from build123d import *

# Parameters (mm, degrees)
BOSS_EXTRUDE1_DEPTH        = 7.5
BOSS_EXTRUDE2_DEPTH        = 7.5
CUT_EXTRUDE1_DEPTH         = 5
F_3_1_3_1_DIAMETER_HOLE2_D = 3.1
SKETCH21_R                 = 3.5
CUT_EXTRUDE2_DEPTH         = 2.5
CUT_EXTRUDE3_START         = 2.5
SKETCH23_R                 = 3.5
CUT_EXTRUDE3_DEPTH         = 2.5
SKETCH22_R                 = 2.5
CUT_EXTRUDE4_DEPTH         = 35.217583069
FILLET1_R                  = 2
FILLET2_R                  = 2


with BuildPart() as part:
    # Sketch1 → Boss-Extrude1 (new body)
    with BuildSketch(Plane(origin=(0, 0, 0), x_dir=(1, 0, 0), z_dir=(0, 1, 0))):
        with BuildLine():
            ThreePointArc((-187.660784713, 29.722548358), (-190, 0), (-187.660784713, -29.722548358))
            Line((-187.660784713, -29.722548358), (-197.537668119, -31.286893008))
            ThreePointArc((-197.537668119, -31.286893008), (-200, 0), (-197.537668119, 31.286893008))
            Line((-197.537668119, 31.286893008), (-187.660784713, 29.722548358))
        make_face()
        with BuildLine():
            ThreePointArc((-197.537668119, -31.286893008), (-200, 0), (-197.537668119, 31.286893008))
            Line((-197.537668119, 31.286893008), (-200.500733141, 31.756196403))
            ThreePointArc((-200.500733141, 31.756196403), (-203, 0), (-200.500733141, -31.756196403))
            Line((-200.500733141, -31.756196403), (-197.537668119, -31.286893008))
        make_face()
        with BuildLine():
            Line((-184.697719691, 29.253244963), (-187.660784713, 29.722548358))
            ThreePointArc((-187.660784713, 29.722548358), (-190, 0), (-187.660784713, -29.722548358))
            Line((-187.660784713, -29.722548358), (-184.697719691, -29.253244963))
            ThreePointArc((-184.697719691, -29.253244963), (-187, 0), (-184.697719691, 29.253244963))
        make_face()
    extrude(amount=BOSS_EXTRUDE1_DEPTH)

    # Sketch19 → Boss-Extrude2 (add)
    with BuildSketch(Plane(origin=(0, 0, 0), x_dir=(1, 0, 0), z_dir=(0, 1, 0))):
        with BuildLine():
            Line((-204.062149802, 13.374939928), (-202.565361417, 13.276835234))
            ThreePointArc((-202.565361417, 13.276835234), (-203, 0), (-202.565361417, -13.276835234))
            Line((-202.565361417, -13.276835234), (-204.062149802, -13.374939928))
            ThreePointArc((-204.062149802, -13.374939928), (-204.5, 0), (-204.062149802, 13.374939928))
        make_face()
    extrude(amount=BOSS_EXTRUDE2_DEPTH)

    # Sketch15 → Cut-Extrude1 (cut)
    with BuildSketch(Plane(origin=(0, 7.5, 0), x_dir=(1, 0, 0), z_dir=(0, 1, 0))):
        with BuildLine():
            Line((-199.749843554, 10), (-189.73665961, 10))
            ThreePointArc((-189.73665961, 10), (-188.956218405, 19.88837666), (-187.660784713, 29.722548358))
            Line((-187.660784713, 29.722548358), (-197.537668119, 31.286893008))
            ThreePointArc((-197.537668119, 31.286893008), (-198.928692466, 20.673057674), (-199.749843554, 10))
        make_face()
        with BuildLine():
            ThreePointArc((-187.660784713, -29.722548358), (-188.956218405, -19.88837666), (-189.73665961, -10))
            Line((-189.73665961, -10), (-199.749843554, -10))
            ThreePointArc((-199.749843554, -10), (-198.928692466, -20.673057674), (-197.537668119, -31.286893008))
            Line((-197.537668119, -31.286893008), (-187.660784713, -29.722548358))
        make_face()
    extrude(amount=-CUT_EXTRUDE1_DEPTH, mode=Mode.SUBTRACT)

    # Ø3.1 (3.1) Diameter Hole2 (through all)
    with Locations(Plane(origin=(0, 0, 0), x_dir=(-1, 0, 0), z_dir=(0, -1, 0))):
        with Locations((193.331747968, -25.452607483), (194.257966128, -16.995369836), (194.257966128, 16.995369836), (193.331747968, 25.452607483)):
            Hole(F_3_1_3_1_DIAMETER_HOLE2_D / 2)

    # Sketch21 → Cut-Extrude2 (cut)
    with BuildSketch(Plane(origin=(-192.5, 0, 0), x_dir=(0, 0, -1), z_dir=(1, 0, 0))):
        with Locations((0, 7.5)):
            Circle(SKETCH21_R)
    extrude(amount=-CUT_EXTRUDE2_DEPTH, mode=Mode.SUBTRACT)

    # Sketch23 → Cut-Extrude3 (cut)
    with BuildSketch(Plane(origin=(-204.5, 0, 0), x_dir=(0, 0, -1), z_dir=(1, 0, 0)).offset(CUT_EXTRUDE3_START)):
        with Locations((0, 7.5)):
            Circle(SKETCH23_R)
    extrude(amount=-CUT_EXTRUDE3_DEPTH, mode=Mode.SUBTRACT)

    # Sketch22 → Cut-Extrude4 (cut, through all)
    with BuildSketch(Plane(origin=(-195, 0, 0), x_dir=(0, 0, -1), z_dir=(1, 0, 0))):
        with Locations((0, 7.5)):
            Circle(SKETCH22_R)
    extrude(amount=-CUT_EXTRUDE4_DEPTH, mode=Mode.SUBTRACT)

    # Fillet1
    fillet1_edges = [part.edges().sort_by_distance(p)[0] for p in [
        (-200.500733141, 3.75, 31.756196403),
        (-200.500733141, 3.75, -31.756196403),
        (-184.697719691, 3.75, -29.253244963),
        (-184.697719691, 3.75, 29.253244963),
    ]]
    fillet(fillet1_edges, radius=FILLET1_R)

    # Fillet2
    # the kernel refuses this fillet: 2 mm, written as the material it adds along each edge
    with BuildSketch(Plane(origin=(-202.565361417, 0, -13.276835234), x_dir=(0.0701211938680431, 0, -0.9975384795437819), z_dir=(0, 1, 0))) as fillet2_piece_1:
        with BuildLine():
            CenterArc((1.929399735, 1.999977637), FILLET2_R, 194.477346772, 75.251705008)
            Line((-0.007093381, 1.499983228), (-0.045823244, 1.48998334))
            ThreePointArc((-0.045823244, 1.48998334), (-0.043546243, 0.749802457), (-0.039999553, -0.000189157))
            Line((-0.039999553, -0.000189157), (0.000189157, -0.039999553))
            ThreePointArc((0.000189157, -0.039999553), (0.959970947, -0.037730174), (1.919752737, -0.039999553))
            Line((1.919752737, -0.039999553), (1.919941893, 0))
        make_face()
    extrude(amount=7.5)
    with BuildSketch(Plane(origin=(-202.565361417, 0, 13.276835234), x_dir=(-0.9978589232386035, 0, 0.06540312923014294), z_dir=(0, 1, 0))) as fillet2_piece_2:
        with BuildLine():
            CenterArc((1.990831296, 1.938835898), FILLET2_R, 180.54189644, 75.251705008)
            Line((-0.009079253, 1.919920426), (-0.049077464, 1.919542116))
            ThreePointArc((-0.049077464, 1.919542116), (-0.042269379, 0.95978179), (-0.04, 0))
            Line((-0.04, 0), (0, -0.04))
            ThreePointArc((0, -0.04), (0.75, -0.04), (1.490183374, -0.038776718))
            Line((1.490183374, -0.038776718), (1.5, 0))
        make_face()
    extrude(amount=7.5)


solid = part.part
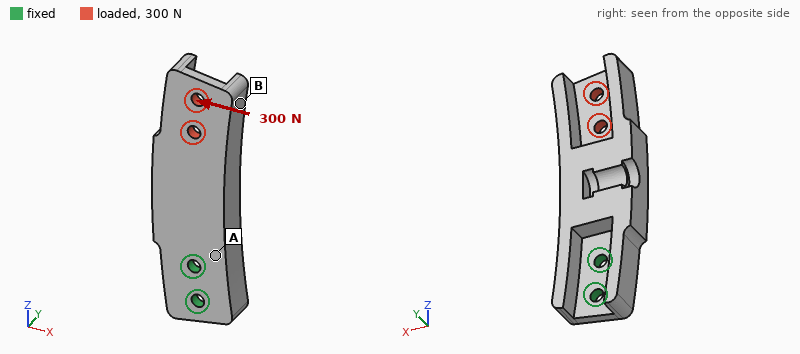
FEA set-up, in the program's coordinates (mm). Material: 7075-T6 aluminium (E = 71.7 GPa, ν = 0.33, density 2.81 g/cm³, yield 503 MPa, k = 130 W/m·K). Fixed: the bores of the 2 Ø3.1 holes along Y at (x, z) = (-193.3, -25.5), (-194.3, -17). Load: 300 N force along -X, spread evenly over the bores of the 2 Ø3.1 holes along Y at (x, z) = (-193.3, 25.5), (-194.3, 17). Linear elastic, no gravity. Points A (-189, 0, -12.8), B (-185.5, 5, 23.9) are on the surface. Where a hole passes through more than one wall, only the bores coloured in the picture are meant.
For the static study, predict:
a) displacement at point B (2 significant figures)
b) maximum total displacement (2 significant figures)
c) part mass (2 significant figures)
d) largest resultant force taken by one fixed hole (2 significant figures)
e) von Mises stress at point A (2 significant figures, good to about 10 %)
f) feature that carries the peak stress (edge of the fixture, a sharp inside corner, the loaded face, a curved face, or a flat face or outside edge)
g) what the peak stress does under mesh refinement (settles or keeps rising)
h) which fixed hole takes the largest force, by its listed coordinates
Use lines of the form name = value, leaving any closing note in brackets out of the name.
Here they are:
displacement at point B = 0.10 mm
maximum total displacement = 0.12 mm
part mass = 15 g
largest resultant force taken by one fixed hole = 1.2 kN
von Mises stress at point A = 39 MPa
feature that carries the peak stress = edge of the fixture
what the peak stress does under mesh refinement = keeps rising
which fixed hole takes the largest force, by its listed coordinates = (-194.3, -17)
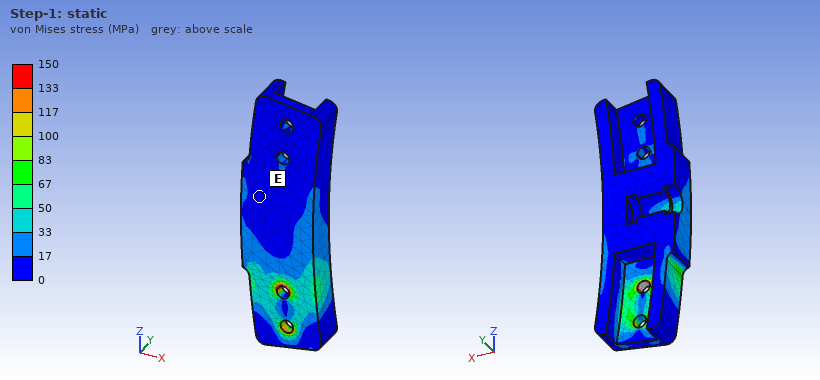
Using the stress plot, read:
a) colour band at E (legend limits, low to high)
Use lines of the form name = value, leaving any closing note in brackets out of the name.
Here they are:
colour band at E = 0 to 17 MPa
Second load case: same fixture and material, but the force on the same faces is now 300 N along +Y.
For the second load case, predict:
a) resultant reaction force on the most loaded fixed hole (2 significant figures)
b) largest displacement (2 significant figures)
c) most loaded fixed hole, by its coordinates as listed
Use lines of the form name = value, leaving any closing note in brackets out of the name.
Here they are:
resultant reaction force on the most loaded fixed hole = 1.2 kN
largest displacement = 0.51 mm
most loaded fixed hole, by its coordinates as listed = (-194.3, -17)
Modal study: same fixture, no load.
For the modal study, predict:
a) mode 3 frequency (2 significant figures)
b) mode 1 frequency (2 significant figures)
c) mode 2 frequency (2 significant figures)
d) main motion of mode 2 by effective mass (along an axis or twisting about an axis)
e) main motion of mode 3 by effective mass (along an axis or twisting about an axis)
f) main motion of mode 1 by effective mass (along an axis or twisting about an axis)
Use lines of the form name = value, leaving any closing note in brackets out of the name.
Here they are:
mode 3 frequency = 5800 Hz
mode 1 frequency = 2000 Hz
mode 2 frequency = 3900 Hz
main motion of mode 2 by effective mass = along X
main motion of mode 3 by effective mass = twisting about Z
main motion of mode 1 by effective mass = along Y
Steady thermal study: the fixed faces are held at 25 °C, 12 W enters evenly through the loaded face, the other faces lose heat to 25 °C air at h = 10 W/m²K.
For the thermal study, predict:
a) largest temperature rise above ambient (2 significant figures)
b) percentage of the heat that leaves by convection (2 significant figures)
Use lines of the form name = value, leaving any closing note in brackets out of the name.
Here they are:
largest temperature rise above ambient = 48 K
percentage of the heat that leaves by convection = 6.4 %
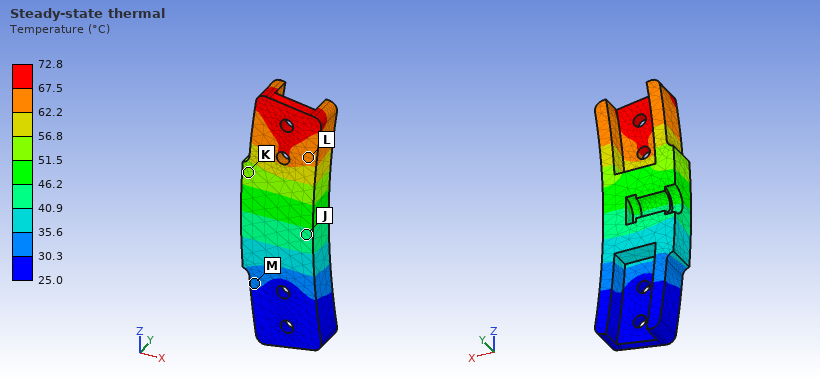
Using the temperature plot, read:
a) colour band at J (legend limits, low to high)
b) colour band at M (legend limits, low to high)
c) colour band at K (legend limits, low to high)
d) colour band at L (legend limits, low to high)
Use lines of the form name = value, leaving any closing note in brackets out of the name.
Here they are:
colour band at J = 40.9 to 46.2 °C
colour band at M = 30.3 to 35.6 °C
colour band at K = 51.5 to 56.8 °C
colour band at L = 62.2 to 67.5 °C
